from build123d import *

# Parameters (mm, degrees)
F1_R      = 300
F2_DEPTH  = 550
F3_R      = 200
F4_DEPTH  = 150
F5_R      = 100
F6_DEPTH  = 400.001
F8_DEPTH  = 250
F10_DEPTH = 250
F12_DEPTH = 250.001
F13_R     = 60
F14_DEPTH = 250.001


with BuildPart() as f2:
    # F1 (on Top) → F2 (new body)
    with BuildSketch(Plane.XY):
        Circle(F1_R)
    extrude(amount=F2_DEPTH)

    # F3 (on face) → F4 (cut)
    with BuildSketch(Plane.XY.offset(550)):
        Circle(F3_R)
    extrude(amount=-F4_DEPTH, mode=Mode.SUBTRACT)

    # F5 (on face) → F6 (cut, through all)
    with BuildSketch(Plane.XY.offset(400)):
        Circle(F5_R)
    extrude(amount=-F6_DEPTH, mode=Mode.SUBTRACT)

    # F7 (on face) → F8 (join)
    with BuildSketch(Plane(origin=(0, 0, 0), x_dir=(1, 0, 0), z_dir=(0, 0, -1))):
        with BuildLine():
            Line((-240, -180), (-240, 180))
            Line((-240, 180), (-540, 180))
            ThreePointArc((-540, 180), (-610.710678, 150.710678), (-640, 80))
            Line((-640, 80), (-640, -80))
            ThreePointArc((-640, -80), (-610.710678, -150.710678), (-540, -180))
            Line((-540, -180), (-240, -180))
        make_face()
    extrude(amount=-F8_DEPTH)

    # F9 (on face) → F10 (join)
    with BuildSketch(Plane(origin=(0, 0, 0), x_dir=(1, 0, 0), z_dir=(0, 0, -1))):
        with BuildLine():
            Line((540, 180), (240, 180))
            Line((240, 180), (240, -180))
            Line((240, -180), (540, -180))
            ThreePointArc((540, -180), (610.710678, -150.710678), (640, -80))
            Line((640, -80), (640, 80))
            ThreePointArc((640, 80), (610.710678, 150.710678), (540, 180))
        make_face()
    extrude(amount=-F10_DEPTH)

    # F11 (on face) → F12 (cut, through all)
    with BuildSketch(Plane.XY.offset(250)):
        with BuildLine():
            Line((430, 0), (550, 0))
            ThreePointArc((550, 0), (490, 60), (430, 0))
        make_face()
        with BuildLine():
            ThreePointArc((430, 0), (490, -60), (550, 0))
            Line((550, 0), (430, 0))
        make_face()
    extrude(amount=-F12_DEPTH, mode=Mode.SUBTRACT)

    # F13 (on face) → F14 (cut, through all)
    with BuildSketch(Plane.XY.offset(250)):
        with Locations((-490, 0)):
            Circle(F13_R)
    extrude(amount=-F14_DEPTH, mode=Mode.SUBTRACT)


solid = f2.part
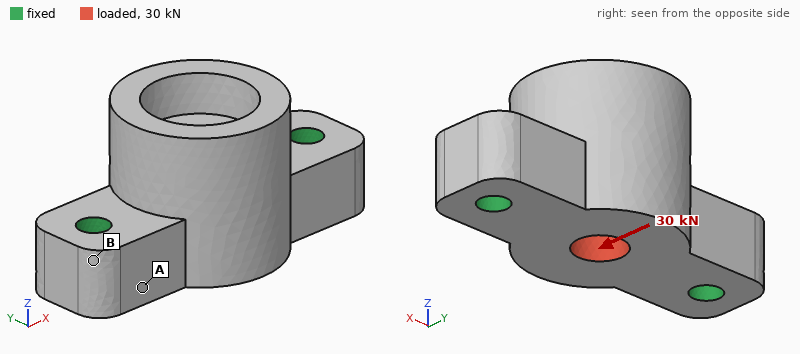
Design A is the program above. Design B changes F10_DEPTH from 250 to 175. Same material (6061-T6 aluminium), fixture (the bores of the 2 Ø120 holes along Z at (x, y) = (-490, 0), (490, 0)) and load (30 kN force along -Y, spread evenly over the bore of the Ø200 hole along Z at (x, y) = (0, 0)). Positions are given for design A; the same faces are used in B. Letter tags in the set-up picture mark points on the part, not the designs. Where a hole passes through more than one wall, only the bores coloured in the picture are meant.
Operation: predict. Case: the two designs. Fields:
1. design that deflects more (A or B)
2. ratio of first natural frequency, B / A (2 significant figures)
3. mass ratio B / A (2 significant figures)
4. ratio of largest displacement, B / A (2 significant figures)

B
0.83
0.95
1.6
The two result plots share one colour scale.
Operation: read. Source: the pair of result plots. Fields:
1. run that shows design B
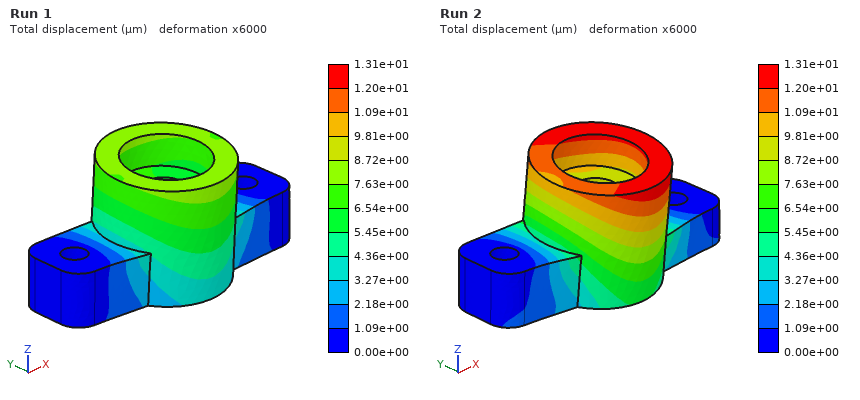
Run 2
